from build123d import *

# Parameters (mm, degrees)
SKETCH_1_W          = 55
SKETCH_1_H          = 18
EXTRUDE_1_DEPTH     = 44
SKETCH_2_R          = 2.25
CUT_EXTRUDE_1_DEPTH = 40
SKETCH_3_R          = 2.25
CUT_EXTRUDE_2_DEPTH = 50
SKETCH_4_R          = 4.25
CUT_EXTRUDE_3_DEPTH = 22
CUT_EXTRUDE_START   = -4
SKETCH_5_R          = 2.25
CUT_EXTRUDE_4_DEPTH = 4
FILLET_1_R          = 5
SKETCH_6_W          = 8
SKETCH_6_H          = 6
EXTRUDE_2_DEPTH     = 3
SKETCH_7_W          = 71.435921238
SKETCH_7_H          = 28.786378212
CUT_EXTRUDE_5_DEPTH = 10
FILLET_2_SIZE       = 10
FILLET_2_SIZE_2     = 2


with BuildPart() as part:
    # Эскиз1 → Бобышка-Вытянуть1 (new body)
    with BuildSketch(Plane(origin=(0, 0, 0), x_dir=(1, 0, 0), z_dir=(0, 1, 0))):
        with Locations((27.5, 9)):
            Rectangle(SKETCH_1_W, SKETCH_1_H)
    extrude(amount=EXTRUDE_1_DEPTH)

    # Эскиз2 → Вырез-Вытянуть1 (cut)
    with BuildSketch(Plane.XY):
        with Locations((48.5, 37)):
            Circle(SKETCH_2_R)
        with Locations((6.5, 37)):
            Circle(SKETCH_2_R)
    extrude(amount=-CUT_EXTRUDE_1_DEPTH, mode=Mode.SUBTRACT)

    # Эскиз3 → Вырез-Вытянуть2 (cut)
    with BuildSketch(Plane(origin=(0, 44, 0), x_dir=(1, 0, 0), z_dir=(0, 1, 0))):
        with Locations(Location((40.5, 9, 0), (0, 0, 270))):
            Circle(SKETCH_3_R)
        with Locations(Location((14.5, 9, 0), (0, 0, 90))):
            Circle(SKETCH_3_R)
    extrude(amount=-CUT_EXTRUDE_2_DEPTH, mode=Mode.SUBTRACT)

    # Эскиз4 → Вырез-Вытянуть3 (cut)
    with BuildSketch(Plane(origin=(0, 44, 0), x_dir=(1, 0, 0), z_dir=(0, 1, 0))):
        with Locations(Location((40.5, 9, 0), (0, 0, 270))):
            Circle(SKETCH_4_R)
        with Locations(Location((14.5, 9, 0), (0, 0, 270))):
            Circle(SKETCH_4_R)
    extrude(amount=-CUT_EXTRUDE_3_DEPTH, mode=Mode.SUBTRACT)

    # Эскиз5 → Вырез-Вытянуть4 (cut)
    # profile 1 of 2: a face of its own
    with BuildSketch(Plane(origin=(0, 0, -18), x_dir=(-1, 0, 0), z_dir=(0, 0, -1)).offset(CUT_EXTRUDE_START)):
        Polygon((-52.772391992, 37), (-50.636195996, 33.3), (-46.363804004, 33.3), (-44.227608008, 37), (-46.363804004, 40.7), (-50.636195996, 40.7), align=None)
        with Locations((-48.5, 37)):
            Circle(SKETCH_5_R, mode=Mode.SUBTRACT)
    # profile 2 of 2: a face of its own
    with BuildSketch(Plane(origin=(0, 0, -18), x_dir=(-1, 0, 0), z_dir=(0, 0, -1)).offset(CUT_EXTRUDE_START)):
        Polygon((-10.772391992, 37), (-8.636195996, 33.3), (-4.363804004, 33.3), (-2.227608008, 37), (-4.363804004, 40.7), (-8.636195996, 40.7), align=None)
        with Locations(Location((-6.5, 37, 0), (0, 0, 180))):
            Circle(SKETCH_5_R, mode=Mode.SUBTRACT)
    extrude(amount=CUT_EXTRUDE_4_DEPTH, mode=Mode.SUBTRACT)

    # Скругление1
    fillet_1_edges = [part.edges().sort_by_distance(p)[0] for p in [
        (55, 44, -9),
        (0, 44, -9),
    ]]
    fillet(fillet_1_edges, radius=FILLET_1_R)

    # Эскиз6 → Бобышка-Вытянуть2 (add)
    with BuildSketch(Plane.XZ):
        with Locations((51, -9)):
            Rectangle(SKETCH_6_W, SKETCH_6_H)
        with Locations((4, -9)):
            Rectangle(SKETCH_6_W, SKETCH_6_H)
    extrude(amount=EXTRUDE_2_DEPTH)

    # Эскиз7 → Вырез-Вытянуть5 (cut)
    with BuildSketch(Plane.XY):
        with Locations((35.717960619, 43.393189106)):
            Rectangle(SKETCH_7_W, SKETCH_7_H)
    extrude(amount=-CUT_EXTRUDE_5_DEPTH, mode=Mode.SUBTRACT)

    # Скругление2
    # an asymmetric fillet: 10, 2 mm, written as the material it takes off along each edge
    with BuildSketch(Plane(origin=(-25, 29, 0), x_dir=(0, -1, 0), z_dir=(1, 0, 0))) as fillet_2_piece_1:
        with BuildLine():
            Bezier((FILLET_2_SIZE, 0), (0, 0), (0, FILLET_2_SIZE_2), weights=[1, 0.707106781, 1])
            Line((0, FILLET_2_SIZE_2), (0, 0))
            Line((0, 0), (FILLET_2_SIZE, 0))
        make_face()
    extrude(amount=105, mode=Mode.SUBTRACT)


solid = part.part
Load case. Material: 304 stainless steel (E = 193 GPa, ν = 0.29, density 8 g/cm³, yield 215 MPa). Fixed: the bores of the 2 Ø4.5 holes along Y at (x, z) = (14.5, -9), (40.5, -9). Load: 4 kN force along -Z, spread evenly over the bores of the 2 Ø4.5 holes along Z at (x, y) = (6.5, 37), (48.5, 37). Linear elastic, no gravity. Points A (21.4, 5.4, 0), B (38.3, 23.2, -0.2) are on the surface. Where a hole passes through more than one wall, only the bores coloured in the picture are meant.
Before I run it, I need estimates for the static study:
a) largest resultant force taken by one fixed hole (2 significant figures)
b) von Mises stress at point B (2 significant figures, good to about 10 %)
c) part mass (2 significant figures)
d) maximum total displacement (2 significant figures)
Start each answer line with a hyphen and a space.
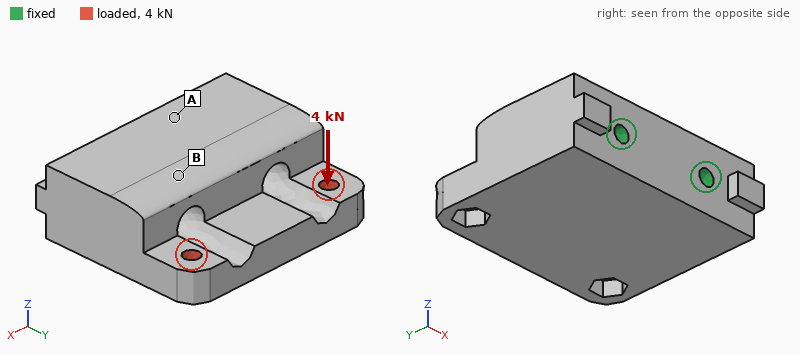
- 2.0 kN
- 19 MPa
- 260 g
- 28 µm
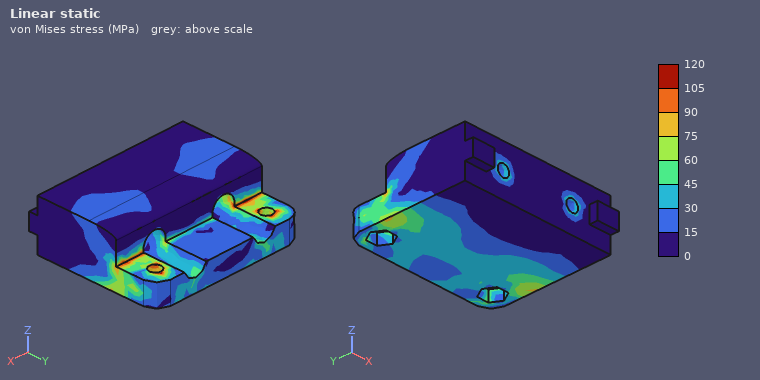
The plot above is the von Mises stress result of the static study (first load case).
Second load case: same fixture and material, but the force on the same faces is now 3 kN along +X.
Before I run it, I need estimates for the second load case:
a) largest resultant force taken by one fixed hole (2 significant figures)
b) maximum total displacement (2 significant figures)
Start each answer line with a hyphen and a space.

- 2.2 kN
- 7.4 µm
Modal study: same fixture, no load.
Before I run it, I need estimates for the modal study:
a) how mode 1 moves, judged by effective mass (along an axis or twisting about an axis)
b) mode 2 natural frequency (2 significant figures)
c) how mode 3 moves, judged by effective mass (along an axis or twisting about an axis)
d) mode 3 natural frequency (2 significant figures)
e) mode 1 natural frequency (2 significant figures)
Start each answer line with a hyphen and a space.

- along Z
- 16 kHz
- along X
- 21 kHz
- 12 kHz
